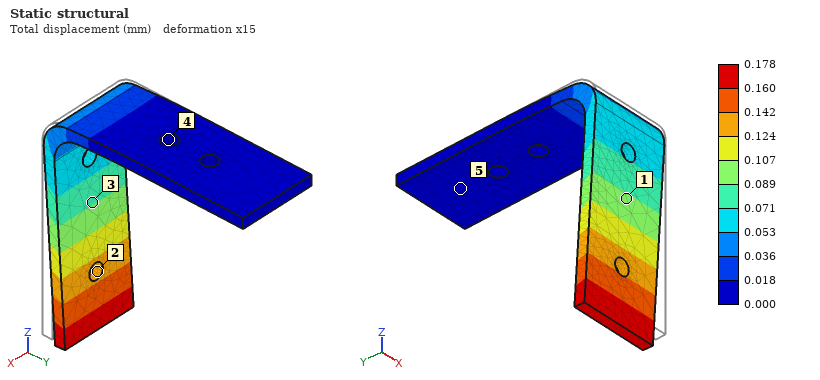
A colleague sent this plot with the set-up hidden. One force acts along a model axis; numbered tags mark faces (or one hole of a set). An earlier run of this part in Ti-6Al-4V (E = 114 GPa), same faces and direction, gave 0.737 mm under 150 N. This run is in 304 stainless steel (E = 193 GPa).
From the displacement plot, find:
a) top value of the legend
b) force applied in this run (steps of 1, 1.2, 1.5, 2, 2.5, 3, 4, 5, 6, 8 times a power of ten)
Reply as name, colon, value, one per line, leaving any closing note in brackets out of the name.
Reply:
top value of the legend: 0.178 mm
force applied in this run: 60 N
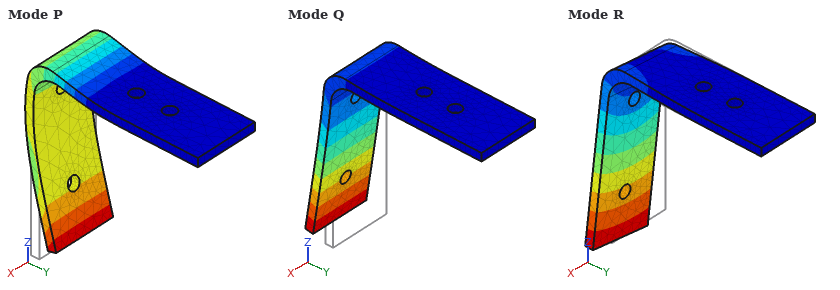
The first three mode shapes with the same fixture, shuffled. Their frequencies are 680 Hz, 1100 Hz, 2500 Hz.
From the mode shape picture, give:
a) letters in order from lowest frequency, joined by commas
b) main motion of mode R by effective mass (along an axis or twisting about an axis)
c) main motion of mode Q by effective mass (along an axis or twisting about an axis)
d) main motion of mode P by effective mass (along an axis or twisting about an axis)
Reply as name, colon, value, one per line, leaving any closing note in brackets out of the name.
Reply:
letters in order from lowest frequency, joined by commas: Q, R, P
main motion of mode R by effective mass: along X
main motion of mode Q by effective mass: along Y
main motion of mode P by effective mass: along Z
